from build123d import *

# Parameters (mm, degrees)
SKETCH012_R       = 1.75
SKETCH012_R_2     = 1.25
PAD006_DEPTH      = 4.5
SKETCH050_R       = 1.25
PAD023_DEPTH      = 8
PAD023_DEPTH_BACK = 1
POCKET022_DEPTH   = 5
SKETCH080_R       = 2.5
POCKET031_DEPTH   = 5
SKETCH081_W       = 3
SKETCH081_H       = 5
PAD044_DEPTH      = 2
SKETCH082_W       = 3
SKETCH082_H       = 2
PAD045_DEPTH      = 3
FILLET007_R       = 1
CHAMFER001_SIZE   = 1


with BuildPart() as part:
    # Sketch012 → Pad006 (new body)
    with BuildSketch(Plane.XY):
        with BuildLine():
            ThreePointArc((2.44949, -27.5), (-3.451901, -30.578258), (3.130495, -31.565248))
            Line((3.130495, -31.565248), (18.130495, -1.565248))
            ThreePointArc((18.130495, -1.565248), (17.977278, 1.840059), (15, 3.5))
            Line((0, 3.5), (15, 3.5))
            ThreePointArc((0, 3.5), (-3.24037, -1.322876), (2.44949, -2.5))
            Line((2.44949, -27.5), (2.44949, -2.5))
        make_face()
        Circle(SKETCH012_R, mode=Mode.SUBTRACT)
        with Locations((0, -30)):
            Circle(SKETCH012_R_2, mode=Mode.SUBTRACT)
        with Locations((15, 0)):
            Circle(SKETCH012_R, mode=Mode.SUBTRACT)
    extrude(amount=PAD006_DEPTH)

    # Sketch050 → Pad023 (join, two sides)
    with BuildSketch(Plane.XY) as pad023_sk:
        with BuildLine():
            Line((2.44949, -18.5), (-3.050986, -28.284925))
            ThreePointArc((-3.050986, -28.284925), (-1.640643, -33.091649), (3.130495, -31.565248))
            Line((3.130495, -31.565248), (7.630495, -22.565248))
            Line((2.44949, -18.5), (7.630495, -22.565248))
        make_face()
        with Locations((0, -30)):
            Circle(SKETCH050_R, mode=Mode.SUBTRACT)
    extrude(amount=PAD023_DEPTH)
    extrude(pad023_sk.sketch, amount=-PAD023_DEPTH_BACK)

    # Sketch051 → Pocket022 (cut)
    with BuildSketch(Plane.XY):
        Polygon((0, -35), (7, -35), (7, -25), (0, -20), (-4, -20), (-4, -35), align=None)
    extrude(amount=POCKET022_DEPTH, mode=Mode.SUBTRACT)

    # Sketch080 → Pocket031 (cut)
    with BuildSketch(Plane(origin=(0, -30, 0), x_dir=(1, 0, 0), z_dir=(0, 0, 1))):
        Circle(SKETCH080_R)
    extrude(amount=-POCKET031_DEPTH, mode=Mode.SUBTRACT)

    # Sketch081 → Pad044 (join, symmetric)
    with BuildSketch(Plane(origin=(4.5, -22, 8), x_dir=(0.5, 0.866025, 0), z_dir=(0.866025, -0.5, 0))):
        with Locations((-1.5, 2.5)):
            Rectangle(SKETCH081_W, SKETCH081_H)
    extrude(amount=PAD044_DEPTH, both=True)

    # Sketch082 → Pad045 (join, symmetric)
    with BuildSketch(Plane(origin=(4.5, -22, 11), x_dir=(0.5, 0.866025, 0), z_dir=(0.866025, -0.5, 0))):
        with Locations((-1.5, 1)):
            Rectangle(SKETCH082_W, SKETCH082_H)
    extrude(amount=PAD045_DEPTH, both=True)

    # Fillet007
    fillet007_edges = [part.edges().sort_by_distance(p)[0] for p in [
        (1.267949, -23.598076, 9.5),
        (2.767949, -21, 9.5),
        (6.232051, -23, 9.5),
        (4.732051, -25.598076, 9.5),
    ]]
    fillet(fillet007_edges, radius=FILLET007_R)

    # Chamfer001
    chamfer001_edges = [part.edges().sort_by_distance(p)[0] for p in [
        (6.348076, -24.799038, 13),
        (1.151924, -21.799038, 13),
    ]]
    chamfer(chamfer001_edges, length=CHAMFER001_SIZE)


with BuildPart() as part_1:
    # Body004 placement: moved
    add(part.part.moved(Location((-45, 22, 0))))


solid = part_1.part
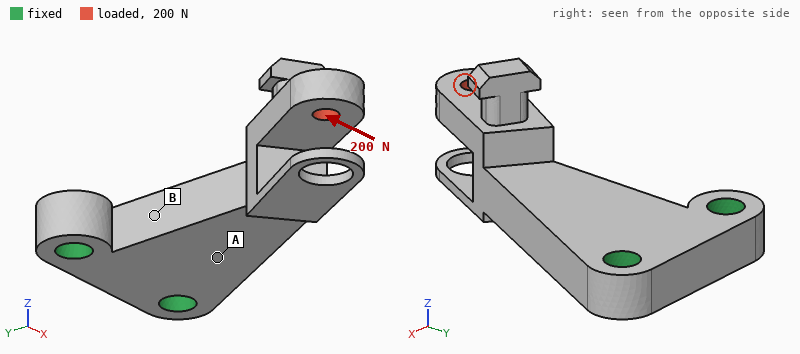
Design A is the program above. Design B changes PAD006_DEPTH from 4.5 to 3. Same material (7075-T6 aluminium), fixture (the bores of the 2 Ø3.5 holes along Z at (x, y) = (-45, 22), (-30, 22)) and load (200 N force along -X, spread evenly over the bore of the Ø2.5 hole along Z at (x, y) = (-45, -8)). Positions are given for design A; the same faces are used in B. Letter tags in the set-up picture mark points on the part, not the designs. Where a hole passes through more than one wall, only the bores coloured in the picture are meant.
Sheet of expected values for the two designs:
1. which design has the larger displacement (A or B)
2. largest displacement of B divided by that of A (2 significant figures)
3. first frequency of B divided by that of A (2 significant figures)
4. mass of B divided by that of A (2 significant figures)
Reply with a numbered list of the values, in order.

1. B
2. 1.9
3. 0.58
4. 0.75
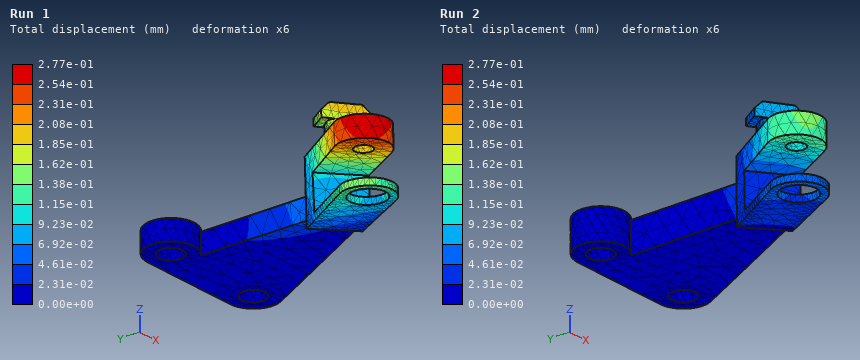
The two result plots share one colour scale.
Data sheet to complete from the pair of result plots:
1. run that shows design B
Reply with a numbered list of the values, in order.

1. Run 1
